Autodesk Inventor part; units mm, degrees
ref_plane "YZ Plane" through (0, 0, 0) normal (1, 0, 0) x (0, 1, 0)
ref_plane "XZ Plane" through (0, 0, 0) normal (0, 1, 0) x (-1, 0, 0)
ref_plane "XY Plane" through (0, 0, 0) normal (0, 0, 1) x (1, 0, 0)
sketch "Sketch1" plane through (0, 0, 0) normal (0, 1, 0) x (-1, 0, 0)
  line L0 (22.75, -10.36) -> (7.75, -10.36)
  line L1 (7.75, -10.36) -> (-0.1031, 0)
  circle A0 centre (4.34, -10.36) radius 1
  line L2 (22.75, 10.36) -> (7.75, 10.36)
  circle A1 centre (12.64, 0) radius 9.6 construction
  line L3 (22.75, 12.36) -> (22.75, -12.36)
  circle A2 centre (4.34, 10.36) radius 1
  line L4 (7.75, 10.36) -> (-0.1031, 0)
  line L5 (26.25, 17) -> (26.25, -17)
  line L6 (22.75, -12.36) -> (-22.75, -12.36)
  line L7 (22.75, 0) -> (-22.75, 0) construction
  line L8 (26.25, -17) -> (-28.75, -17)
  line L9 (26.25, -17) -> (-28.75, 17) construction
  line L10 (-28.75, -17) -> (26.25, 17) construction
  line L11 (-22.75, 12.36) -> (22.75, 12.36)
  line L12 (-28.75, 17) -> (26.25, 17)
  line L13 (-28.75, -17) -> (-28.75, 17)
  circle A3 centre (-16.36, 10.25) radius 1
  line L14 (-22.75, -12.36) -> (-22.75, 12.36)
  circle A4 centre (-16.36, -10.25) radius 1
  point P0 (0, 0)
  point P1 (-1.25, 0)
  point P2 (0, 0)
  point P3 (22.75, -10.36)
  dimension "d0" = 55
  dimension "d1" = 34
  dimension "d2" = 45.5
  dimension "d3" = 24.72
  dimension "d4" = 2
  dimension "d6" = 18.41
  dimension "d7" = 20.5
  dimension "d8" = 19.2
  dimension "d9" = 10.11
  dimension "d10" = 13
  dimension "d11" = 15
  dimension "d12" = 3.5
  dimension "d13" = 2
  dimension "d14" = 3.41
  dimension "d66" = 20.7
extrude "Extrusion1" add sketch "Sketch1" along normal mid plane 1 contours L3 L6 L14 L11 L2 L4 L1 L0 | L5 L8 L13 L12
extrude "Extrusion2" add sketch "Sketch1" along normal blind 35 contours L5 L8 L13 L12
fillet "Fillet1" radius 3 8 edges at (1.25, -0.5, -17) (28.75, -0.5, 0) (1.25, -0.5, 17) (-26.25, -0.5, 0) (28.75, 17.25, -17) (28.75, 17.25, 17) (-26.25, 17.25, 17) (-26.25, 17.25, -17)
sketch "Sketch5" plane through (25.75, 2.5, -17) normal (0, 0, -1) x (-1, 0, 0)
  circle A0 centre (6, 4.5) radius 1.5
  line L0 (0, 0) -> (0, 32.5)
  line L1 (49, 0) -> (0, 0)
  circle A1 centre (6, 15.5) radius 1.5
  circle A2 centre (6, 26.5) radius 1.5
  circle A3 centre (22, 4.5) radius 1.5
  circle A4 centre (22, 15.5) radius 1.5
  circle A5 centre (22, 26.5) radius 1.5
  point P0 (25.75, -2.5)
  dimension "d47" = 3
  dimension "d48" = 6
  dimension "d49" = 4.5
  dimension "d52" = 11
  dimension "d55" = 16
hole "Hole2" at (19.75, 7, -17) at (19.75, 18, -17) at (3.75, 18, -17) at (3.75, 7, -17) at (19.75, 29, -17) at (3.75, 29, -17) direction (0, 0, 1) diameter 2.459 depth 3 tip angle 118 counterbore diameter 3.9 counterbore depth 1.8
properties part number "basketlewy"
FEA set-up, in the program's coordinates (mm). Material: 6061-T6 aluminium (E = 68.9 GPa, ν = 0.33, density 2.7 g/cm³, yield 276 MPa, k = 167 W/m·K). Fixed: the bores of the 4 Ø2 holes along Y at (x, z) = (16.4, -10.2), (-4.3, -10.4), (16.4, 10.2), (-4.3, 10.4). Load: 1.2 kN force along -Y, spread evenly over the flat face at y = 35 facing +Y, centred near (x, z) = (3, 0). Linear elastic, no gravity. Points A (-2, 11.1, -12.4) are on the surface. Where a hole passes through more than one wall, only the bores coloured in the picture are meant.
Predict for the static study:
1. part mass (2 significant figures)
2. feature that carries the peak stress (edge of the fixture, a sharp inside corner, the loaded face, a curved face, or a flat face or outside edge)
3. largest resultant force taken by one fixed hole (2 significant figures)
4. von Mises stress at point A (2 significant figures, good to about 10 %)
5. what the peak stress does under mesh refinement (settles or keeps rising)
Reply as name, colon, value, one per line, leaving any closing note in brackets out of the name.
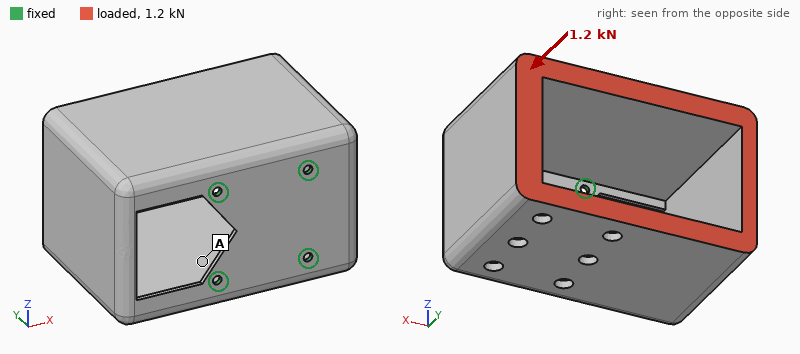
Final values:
part mass: 71 g
feature that carries the peak stress: edge of the fixture
largest resultant force taken by one fixed hole: 390 N
von Mises stress at point A: 8.7 MPa
what the peak stress does under mesh refinement: keeps rising
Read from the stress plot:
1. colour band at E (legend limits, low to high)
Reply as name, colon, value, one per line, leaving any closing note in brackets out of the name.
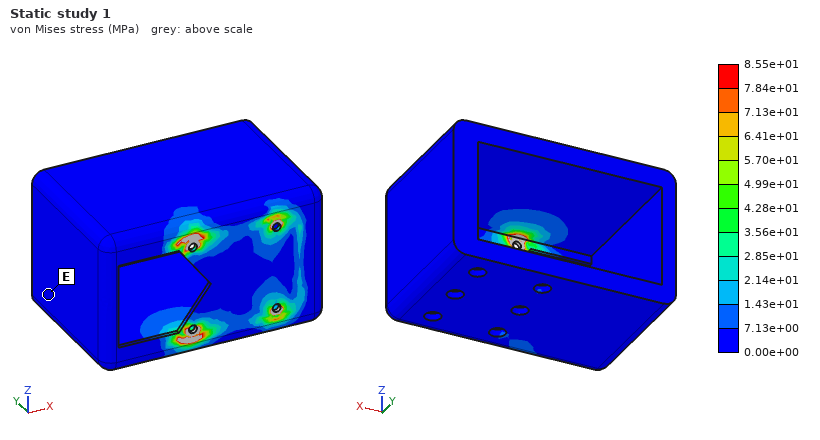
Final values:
colour band at E: 0.00e+00 to 7.13e+00 MPa
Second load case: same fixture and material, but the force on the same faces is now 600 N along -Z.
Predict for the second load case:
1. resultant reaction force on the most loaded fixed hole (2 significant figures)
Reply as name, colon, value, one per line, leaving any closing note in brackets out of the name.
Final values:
resultant reaction force on the most loaded fixed hole: 530 N
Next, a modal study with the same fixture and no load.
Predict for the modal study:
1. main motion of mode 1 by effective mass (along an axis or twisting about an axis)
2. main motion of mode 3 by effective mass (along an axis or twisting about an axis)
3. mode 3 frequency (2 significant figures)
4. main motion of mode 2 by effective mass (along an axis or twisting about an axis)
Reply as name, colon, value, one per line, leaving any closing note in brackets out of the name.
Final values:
main motion of mode 1 by effective mass: along Z
main motion of mode 3 by effective mass: twisting about Y
mode 3 frequency: 4100 Hz
main motion of mode 2 by effective mass: along X
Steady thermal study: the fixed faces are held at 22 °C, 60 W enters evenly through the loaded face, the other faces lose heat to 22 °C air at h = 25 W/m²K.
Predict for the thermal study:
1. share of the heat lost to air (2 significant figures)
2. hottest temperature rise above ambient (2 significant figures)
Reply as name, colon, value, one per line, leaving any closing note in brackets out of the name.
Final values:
share of the heat lost to air: 17 %
hottest temperature rise above ambient: 44 K
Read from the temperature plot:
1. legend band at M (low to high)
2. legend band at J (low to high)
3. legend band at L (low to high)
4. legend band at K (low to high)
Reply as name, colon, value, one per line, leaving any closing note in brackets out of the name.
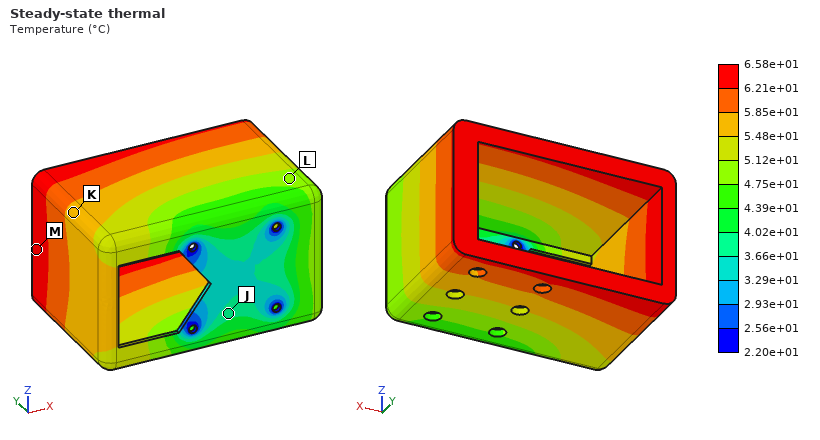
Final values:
legend band at M: 6.21e+01 to 6.58e+01 °C
legend band at J: 3.66e+01 to 4.02e+01 °C
legend band at L: 4.75e+01 to 5.12e+01 °C
legend band at K: 5.48e+01 to 5.85e+01 °C
